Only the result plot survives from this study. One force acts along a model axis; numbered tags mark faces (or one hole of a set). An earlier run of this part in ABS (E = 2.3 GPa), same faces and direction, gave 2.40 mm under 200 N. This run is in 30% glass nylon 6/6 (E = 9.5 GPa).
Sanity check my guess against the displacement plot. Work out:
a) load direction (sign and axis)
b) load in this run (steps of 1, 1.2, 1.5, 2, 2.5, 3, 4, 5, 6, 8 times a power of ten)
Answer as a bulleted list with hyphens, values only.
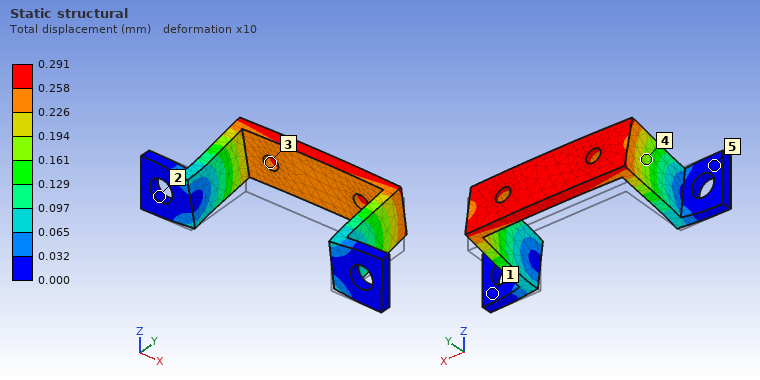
- +Z
- 100 N
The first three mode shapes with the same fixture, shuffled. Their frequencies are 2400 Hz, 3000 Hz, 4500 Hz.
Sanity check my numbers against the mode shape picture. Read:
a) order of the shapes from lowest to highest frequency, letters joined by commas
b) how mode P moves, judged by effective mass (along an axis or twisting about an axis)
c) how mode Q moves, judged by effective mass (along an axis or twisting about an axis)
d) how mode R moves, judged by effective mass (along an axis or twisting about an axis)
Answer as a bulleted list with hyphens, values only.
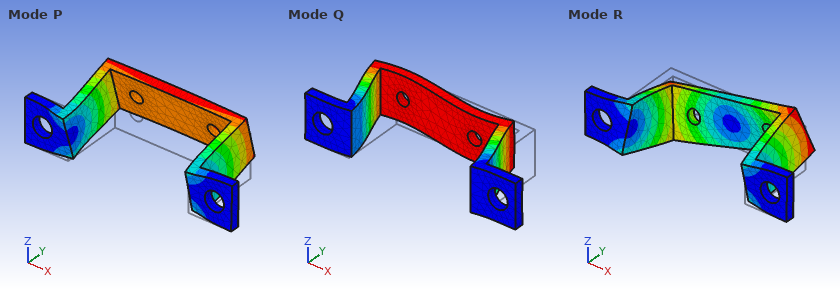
- Q, P, R
- along Z
- along X
- twisting about Y
